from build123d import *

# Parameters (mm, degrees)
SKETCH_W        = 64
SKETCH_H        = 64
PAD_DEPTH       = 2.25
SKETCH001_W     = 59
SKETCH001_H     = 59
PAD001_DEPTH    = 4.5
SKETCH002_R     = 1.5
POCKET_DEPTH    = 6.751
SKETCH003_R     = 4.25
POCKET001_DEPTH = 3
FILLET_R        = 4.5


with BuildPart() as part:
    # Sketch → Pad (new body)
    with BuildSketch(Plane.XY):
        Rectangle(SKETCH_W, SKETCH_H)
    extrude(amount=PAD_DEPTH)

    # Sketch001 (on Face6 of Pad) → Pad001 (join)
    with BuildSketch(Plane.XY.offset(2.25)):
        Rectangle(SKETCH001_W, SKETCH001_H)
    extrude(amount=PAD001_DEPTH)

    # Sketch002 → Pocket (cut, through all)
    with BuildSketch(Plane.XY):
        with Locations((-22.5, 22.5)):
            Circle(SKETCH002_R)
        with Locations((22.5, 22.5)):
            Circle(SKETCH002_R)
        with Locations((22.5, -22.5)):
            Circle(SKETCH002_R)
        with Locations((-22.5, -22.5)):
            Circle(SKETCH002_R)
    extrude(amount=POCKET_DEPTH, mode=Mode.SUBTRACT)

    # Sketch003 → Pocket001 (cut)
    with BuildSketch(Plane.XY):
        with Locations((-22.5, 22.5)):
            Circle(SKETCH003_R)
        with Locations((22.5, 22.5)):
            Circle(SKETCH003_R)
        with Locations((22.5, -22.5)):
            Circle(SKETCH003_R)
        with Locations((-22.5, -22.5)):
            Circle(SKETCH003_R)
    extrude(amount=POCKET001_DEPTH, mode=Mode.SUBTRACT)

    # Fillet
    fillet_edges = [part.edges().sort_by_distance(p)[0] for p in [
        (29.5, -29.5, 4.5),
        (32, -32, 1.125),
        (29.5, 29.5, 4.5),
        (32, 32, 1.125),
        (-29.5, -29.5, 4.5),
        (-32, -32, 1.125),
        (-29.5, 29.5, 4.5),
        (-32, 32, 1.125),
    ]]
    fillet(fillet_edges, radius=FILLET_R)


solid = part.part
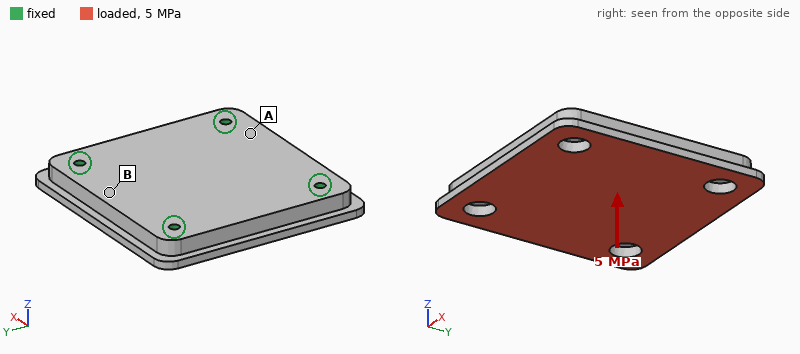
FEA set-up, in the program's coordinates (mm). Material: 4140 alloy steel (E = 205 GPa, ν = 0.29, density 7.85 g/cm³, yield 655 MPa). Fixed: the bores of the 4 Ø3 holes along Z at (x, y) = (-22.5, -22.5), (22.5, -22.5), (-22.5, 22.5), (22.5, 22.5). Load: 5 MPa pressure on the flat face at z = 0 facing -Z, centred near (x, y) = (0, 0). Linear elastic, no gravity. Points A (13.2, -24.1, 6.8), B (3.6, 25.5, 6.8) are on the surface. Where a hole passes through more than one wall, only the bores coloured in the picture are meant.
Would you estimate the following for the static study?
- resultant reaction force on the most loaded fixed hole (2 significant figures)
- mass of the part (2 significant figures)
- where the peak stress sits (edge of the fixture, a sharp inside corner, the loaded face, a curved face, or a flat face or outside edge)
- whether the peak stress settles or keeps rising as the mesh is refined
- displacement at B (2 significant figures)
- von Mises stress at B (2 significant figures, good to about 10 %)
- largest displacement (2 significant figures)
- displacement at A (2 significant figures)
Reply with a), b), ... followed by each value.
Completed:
a) 5.5 kN
b) 190 g
c) edge of the fixture
d) keeps rising
e) 28 µm
f) 91 MPa
g) 47 µm
h) 18 µm
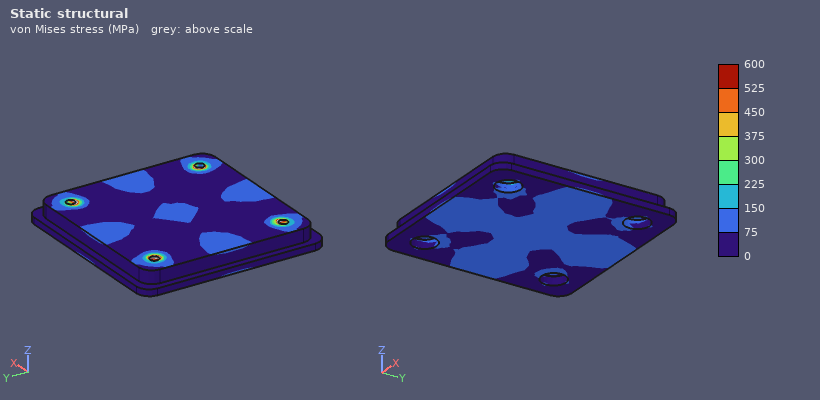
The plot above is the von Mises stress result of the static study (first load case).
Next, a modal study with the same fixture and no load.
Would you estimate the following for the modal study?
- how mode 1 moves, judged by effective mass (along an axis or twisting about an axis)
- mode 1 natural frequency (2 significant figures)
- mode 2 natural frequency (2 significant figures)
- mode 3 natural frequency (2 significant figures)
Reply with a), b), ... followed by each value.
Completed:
a) along Z
b) 8400 Hz
c) 12 kHz
d) 13 kHz
